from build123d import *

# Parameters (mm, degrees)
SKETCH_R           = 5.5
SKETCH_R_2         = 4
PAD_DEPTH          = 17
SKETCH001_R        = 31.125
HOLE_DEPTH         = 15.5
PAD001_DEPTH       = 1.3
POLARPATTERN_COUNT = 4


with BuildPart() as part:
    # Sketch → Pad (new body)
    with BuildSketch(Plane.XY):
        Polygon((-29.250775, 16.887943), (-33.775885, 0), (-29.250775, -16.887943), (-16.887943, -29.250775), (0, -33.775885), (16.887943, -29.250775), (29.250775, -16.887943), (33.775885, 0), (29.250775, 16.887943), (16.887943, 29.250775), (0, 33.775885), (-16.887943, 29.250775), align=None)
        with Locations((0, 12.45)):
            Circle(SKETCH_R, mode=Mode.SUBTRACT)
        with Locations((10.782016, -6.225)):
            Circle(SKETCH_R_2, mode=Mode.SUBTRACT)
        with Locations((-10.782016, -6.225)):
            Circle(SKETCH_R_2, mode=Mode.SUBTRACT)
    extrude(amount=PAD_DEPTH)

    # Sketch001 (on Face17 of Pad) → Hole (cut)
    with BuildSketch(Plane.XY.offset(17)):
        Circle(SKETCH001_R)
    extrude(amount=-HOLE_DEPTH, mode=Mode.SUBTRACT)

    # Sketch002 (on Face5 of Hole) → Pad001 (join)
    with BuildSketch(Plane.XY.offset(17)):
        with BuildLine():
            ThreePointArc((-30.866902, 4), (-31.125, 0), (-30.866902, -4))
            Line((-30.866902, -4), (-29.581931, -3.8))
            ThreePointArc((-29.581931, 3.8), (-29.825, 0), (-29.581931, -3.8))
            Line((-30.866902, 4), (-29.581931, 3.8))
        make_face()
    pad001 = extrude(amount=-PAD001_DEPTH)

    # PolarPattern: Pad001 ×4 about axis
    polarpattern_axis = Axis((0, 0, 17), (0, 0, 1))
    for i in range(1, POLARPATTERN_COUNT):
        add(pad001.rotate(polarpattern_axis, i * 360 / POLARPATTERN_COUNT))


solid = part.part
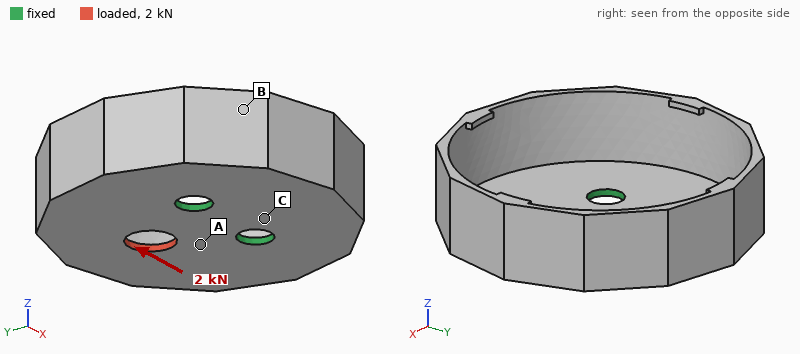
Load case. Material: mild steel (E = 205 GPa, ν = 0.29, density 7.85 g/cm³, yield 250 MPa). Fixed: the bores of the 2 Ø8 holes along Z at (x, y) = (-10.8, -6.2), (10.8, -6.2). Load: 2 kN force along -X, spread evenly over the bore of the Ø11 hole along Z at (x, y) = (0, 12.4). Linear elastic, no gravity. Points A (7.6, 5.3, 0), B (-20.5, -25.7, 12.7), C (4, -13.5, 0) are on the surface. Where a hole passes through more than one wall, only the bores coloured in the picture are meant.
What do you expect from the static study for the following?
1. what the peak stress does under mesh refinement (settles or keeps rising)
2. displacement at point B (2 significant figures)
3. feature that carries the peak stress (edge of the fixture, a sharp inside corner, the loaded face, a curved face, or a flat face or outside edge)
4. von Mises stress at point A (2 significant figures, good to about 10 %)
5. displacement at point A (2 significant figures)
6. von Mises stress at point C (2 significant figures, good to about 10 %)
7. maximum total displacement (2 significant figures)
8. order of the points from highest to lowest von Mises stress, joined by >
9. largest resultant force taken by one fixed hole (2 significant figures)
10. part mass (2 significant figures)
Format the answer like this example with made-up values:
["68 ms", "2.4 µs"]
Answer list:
["keeps rising", "4.1 µm", "edge of the fixture", "48 MPa", "4.8 µm", "19 MPa", "17 µm", "A > C > B", "1.5 kN", "85 g"]
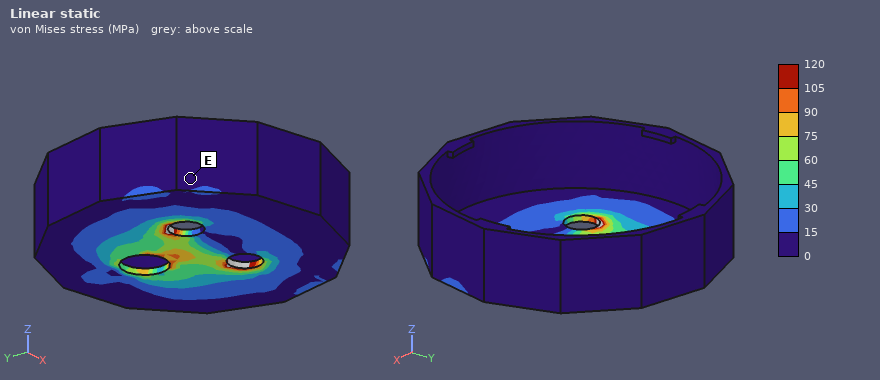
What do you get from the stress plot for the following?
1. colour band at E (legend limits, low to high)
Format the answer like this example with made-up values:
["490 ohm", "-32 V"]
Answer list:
["0 to 15 MPa"]
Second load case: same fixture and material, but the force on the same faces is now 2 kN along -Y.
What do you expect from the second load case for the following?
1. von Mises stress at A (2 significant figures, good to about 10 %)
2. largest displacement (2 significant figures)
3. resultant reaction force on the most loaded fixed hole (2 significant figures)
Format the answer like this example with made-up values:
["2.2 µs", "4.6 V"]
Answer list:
["47 MPa", "5.7 µm", "1.0 kN"]
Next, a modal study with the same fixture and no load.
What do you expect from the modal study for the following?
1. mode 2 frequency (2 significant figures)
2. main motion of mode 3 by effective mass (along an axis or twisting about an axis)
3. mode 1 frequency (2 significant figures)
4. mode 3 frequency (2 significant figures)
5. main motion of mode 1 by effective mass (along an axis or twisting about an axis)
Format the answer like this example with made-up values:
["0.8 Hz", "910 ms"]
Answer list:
["1700 Hz", "along Z", "850 Hz", "2300 Hz", "along Z"]
